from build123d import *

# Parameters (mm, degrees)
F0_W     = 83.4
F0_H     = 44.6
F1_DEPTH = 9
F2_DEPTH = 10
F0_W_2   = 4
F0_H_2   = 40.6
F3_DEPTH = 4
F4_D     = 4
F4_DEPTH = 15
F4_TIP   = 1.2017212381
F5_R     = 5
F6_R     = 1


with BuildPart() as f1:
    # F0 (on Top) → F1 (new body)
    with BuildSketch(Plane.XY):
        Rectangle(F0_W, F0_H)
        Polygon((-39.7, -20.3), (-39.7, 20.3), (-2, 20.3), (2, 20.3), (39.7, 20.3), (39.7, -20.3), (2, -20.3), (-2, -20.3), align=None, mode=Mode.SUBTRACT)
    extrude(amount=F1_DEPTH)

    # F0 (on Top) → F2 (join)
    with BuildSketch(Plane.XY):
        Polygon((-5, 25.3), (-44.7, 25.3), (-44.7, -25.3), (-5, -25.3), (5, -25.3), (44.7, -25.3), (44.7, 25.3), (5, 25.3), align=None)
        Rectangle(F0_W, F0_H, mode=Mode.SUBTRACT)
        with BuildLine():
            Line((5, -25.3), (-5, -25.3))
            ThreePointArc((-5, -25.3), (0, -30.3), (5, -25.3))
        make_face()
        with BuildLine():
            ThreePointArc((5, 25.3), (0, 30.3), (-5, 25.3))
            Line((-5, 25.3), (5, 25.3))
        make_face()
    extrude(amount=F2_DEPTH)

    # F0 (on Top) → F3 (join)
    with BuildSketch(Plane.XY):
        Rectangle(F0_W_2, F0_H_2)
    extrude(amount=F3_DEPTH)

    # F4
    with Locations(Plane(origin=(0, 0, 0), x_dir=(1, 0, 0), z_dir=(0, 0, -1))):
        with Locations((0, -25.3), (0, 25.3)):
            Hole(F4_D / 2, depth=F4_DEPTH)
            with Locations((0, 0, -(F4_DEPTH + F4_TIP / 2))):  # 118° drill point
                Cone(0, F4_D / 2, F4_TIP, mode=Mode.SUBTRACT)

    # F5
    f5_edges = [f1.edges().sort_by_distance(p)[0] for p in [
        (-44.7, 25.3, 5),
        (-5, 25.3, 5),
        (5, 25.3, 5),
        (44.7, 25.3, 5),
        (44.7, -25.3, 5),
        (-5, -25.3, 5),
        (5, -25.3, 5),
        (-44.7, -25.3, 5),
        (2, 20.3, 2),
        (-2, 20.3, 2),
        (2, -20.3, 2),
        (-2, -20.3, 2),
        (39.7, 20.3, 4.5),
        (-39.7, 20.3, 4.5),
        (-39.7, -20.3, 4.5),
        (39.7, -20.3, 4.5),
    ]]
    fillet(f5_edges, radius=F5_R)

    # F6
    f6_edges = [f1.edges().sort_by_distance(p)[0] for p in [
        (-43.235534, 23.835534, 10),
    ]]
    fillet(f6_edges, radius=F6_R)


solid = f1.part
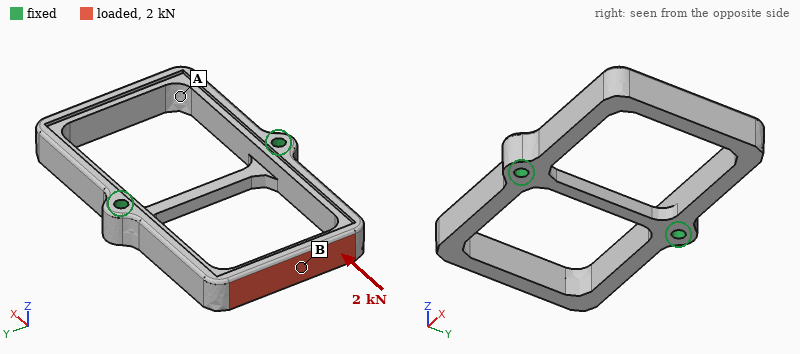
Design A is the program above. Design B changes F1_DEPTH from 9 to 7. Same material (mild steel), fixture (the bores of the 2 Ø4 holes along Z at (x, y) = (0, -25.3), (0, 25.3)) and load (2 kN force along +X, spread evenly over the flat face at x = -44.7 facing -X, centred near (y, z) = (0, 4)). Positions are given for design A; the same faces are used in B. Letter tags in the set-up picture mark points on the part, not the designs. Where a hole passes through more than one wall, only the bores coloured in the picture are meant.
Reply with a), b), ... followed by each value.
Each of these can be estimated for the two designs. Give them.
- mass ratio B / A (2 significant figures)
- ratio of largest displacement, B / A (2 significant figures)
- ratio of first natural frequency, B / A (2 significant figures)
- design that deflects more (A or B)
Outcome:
a) 0.92
b) 1.3
c) 0.96
d) B
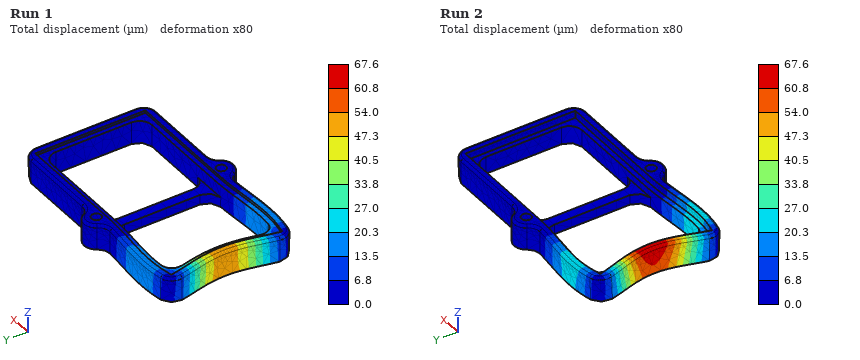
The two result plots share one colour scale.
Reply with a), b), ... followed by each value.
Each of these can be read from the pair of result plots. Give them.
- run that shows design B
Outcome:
a) Run 2
